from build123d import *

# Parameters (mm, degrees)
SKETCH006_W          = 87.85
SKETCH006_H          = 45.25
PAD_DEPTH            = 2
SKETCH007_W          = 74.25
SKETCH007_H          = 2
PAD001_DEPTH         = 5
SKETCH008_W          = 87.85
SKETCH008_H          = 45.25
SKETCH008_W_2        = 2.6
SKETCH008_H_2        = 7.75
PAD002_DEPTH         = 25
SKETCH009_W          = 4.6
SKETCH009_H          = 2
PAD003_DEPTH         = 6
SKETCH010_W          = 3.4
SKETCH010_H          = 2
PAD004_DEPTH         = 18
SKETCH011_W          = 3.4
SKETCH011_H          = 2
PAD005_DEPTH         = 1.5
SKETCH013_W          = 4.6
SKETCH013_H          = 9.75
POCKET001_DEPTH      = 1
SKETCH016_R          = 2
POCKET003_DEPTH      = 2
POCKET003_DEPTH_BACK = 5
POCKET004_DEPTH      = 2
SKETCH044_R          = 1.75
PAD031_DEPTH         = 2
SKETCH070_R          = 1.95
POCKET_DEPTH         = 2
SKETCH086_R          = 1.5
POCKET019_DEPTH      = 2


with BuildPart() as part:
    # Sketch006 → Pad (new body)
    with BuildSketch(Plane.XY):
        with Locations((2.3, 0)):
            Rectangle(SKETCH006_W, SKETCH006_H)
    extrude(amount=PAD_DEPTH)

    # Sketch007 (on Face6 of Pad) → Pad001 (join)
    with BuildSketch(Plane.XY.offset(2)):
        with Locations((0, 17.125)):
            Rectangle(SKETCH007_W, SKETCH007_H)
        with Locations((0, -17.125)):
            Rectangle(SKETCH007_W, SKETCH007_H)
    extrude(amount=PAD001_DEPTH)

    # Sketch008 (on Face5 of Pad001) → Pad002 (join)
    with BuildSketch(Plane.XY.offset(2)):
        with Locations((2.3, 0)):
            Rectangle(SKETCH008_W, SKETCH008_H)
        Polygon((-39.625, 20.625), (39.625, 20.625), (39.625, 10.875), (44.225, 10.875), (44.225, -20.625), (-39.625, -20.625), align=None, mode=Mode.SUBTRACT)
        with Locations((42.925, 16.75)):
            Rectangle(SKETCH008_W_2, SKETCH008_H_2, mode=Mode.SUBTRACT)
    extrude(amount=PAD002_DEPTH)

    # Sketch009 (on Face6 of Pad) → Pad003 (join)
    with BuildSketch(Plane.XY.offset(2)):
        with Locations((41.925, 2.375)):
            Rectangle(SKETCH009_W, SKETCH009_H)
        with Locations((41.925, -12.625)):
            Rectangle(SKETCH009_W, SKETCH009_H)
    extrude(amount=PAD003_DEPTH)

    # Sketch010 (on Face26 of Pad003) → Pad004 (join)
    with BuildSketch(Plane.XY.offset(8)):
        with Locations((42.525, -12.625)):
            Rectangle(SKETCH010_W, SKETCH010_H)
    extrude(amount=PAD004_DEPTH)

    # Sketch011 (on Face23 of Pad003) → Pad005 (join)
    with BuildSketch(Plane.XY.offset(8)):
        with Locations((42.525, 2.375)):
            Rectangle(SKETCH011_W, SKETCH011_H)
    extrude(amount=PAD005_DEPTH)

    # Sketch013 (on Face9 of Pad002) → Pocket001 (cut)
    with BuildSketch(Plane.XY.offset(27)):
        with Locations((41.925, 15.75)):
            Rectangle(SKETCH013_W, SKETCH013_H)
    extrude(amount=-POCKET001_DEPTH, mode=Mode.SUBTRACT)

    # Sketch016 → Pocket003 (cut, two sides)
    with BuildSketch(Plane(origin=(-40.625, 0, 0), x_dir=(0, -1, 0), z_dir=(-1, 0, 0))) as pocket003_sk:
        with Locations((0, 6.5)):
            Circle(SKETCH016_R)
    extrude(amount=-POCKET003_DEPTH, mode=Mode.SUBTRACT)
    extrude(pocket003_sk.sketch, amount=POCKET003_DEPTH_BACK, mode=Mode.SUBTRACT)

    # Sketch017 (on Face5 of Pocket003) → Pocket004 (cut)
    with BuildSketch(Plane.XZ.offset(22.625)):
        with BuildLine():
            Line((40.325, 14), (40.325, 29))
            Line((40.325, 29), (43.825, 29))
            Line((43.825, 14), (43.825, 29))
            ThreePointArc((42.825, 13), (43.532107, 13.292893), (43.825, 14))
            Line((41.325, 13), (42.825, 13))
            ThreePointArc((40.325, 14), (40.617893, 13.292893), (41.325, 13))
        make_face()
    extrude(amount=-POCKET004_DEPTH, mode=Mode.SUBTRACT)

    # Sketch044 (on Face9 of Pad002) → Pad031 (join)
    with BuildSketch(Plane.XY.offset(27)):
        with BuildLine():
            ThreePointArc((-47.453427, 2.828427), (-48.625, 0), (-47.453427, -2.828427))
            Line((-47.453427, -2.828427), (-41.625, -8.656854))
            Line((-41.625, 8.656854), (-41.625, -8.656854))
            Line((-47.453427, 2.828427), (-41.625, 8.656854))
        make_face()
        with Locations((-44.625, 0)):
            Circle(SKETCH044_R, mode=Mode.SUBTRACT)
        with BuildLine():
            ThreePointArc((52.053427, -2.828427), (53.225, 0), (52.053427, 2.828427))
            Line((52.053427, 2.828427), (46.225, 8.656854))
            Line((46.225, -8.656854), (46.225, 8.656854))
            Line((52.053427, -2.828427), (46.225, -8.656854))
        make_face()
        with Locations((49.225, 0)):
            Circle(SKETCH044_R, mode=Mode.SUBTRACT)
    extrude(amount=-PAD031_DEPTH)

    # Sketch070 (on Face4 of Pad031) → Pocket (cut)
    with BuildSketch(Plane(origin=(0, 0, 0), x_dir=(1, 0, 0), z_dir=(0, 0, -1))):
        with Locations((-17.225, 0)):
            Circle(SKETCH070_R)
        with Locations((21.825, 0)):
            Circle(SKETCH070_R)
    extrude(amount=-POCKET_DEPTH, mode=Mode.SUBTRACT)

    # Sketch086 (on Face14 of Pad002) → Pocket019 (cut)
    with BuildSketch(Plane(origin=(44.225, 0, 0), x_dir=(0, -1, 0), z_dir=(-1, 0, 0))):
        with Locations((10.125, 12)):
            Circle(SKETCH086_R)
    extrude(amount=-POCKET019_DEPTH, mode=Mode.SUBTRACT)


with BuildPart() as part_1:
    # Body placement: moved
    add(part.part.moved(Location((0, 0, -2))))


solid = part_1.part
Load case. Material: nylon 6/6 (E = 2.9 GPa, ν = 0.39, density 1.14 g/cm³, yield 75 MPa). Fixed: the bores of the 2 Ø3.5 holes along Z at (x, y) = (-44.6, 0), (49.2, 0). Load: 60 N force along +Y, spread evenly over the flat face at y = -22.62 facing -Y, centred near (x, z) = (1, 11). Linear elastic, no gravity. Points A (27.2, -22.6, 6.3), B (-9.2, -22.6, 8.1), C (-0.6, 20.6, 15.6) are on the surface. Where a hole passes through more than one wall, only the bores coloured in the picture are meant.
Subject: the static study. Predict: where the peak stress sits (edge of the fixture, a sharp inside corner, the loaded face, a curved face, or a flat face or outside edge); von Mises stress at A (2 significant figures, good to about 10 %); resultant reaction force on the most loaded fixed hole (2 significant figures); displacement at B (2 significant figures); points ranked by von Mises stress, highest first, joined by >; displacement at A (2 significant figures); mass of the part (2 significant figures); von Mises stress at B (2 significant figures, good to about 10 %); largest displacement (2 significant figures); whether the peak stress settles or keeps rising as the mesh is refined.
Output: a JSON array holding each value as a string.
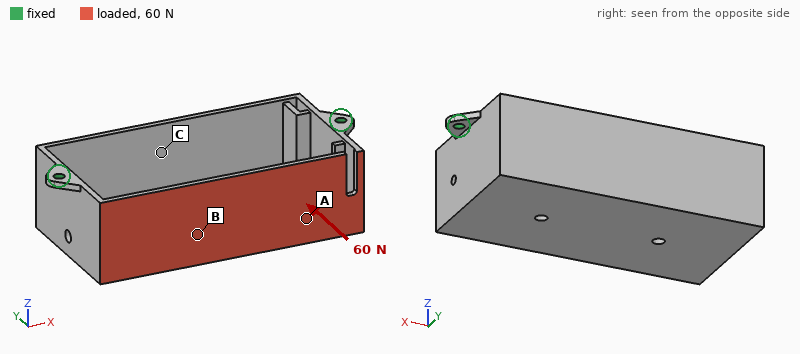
["edge of the fixture", "5.2 MPa", "31 N", "0.73 mm", "A > B > C", "0.73 mm", "26 g", "3.2 MPa", "1.1 mm", "keeps rising"]
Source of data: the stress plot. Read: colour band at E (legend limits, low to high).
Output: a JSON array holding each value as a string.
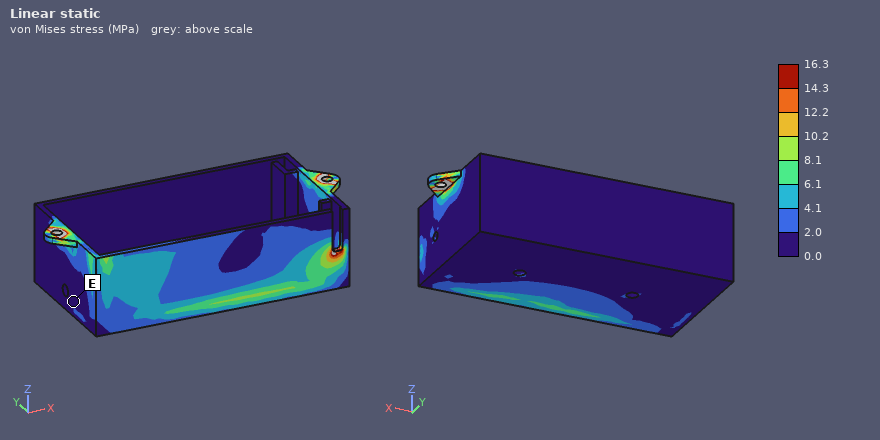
["0.0 to 2.0 MPa"]
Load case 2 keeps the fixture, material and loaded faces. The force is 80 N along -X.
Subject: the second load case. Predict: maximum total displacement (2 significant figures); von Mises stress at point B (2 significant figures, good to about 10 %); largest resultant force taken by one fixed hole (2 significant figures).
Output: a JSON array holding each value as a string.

["1.1 mm", "2.9 MPa", "45 N"]
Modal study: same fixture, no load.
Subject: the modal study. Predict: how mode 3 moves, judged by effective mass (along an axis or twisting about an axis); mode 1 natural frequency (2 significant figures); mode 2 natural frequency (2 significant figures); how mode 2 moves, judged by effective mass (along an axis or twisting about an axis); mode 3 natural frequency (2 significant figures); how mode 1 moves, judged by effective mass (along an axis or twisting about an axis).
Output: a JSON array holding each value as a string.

["along X", "230 Hz", "430 Hz", "along X", "570 Hz", "along Y"]
